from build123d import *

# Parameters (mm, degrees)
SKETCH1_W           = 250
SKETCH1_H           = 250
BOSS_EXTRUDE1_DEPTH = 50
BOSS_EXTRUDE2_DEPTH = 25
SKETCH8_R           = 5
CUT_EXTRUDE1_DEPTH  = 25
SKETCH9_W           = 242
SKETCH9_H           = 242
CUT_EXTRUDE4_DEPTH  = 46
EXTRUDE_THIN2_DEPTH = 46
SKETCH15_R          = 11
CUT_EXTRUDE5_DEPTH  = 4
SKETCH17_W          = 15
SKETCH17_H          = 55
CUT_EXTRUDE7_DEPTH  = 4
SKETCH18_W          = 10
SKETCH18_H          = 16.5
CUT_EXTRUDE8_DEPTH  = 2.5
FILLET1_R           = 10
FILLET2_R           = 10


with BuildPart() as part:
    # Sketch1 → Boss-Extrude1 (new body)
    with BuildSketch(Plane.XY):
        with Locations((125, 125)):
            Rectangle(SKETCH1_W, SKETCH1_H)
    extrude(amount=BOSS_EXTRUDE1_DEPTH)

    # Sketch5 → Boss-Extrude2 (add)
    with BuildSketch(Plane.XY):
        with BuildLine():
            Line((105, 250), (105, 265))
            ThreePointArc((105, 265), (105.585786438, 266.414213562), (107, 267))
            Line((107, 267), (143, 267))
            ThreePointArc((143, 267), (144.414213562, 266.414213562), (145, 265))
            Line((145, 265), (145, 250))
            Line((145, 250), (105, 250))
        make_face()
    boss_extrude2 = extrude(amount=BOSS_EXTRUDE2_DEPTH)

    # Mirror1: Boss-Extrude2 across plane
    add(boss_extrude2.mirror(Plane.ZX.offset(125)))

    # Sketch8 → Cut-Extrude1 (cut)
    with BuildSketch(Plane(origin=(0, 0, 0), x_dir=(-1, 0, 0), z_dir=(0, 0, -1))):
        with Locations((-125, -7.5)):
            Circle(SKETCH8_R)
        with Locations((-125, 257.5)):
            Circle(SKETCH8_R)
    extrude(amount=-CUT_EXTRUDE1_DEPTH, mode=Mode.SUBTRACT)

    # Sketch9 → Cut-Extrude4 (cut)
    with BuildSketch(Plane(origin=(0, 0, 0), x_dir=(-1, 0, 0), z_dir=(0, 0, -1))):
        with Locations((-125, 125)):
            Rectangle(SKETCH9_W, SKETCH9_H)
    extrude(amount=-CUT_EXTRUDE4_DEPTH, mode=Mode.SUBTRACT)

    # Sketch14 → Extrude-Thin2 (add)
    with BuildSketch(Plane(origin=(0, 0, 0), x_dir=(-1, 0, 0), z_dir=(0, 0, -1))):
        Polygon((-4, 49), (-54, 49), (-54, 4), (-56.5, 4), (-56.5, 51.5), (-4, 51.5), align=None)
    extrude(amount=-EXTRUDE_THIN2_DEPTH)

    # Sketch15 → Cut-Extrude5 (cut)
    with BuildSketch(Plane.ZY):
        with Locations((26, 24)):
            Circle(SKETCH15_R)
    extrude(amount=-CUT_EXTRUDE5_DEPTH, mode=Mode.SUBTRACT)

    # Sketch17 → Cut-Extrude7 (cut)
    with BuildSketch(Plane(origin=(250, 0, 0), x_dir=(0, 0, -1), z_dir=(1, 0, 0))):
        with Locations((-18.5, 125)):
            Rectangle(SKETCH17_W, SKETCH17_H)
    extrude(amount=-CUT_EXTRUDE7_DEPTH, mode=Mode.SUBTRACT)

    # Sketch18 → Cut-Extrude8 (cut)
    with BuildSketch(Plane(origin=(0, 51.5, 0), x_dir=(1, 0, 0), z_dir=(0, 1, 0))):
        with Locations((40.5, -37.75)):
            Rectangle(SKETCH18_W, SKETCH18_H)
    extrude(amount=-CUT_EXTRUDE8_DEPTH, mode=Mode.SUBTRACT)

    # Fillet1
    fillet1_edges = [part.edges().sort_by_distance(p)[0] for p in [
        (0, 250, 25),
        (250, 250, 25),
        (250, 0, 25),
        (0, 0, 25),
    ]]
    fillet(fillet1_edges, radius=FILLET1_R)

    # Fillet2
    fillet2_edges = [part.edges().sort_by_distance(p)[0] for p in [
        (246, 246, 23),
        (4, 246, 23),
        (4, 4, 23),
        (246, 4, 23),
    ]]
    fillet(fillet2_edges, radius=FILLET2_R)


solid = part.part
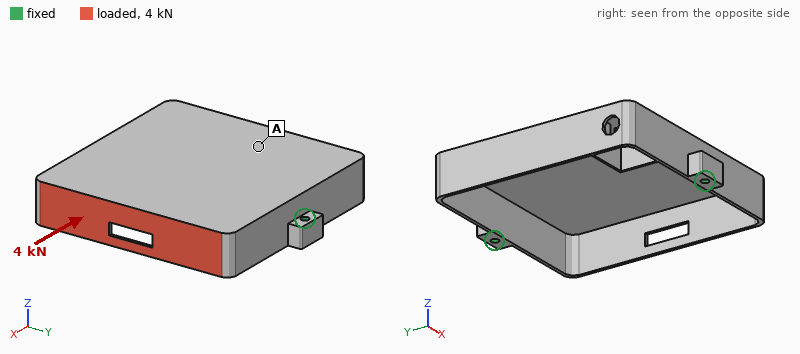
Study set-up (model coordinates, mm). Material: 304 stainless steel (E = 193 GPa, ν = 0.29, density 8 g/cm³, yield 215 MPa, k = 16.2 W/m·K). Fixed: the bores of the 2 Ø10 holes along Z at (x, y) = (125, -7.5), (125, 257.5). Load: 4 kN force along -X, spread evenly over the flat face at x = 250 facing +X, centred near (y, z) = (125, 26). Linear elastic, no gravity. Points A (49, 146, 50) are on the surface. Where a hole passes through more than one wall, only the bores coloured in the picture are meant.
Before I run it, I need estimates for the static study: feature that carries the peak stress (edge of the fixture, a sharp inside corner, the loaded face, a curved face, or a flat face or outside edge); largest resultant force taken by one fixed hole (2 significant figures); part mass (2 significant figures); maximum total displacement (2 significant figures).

the loaded face
2.0 kN
3.7 kg
0.49 mm
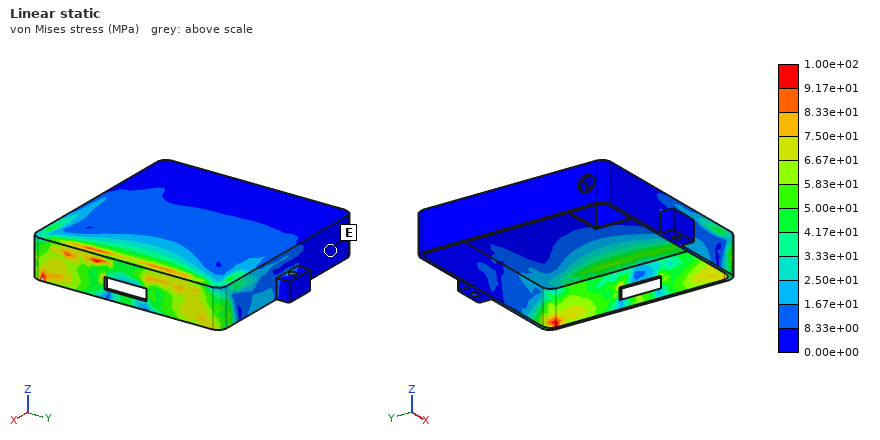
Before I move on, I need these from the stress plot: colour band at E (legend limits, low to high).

0.00e+00 to 8.33e+00 MPa
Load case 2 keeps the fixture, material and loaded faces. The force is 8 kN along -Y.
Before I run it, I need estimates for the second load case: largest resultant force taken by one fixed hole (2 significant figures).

5.7 kN
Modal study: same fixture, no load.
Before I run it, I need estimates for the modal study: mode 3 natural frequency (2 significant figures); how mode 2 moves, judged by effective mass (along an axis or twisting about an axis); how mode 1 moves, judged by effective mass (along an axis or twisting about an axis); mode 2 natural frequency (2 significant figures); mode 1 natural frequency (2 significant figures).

630 Hz
along Y
along Z
610 Hz
460 Hz
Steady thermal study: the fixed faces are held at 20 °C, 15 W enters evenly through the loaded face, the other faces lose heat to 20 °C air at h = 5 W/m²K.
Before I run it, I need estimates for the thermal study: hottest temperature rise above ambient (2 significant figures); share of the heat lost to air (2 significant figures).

68 K
85 %
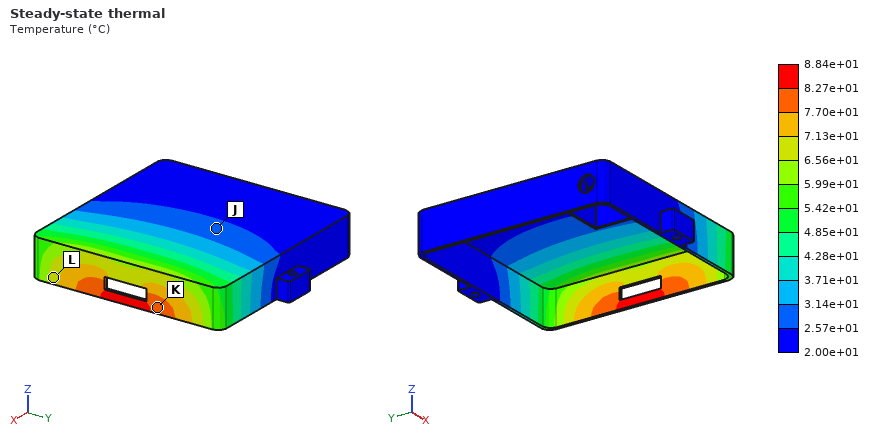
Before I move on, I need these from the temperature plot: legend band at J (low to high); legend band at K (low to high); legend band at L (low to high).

2.57e+01 to 3.14e+01 °C
7.70e+01 to 8.27e+01 °C
6.56e+01 to 7.13e+01 °C
